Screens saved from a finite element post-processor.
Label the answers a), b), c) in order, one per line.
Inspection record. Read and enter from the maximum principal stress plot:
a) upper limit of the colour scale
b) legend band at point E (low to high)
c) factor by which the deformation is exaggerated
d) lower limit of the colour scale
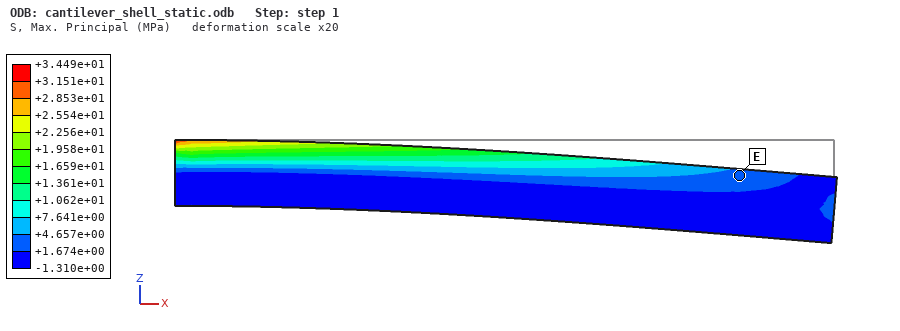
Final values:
a) +3.449e+01 MPa
b) +1.674e+00 to +4.657e+00 MPa
c) 20
d) -1.310e+00 MPa
